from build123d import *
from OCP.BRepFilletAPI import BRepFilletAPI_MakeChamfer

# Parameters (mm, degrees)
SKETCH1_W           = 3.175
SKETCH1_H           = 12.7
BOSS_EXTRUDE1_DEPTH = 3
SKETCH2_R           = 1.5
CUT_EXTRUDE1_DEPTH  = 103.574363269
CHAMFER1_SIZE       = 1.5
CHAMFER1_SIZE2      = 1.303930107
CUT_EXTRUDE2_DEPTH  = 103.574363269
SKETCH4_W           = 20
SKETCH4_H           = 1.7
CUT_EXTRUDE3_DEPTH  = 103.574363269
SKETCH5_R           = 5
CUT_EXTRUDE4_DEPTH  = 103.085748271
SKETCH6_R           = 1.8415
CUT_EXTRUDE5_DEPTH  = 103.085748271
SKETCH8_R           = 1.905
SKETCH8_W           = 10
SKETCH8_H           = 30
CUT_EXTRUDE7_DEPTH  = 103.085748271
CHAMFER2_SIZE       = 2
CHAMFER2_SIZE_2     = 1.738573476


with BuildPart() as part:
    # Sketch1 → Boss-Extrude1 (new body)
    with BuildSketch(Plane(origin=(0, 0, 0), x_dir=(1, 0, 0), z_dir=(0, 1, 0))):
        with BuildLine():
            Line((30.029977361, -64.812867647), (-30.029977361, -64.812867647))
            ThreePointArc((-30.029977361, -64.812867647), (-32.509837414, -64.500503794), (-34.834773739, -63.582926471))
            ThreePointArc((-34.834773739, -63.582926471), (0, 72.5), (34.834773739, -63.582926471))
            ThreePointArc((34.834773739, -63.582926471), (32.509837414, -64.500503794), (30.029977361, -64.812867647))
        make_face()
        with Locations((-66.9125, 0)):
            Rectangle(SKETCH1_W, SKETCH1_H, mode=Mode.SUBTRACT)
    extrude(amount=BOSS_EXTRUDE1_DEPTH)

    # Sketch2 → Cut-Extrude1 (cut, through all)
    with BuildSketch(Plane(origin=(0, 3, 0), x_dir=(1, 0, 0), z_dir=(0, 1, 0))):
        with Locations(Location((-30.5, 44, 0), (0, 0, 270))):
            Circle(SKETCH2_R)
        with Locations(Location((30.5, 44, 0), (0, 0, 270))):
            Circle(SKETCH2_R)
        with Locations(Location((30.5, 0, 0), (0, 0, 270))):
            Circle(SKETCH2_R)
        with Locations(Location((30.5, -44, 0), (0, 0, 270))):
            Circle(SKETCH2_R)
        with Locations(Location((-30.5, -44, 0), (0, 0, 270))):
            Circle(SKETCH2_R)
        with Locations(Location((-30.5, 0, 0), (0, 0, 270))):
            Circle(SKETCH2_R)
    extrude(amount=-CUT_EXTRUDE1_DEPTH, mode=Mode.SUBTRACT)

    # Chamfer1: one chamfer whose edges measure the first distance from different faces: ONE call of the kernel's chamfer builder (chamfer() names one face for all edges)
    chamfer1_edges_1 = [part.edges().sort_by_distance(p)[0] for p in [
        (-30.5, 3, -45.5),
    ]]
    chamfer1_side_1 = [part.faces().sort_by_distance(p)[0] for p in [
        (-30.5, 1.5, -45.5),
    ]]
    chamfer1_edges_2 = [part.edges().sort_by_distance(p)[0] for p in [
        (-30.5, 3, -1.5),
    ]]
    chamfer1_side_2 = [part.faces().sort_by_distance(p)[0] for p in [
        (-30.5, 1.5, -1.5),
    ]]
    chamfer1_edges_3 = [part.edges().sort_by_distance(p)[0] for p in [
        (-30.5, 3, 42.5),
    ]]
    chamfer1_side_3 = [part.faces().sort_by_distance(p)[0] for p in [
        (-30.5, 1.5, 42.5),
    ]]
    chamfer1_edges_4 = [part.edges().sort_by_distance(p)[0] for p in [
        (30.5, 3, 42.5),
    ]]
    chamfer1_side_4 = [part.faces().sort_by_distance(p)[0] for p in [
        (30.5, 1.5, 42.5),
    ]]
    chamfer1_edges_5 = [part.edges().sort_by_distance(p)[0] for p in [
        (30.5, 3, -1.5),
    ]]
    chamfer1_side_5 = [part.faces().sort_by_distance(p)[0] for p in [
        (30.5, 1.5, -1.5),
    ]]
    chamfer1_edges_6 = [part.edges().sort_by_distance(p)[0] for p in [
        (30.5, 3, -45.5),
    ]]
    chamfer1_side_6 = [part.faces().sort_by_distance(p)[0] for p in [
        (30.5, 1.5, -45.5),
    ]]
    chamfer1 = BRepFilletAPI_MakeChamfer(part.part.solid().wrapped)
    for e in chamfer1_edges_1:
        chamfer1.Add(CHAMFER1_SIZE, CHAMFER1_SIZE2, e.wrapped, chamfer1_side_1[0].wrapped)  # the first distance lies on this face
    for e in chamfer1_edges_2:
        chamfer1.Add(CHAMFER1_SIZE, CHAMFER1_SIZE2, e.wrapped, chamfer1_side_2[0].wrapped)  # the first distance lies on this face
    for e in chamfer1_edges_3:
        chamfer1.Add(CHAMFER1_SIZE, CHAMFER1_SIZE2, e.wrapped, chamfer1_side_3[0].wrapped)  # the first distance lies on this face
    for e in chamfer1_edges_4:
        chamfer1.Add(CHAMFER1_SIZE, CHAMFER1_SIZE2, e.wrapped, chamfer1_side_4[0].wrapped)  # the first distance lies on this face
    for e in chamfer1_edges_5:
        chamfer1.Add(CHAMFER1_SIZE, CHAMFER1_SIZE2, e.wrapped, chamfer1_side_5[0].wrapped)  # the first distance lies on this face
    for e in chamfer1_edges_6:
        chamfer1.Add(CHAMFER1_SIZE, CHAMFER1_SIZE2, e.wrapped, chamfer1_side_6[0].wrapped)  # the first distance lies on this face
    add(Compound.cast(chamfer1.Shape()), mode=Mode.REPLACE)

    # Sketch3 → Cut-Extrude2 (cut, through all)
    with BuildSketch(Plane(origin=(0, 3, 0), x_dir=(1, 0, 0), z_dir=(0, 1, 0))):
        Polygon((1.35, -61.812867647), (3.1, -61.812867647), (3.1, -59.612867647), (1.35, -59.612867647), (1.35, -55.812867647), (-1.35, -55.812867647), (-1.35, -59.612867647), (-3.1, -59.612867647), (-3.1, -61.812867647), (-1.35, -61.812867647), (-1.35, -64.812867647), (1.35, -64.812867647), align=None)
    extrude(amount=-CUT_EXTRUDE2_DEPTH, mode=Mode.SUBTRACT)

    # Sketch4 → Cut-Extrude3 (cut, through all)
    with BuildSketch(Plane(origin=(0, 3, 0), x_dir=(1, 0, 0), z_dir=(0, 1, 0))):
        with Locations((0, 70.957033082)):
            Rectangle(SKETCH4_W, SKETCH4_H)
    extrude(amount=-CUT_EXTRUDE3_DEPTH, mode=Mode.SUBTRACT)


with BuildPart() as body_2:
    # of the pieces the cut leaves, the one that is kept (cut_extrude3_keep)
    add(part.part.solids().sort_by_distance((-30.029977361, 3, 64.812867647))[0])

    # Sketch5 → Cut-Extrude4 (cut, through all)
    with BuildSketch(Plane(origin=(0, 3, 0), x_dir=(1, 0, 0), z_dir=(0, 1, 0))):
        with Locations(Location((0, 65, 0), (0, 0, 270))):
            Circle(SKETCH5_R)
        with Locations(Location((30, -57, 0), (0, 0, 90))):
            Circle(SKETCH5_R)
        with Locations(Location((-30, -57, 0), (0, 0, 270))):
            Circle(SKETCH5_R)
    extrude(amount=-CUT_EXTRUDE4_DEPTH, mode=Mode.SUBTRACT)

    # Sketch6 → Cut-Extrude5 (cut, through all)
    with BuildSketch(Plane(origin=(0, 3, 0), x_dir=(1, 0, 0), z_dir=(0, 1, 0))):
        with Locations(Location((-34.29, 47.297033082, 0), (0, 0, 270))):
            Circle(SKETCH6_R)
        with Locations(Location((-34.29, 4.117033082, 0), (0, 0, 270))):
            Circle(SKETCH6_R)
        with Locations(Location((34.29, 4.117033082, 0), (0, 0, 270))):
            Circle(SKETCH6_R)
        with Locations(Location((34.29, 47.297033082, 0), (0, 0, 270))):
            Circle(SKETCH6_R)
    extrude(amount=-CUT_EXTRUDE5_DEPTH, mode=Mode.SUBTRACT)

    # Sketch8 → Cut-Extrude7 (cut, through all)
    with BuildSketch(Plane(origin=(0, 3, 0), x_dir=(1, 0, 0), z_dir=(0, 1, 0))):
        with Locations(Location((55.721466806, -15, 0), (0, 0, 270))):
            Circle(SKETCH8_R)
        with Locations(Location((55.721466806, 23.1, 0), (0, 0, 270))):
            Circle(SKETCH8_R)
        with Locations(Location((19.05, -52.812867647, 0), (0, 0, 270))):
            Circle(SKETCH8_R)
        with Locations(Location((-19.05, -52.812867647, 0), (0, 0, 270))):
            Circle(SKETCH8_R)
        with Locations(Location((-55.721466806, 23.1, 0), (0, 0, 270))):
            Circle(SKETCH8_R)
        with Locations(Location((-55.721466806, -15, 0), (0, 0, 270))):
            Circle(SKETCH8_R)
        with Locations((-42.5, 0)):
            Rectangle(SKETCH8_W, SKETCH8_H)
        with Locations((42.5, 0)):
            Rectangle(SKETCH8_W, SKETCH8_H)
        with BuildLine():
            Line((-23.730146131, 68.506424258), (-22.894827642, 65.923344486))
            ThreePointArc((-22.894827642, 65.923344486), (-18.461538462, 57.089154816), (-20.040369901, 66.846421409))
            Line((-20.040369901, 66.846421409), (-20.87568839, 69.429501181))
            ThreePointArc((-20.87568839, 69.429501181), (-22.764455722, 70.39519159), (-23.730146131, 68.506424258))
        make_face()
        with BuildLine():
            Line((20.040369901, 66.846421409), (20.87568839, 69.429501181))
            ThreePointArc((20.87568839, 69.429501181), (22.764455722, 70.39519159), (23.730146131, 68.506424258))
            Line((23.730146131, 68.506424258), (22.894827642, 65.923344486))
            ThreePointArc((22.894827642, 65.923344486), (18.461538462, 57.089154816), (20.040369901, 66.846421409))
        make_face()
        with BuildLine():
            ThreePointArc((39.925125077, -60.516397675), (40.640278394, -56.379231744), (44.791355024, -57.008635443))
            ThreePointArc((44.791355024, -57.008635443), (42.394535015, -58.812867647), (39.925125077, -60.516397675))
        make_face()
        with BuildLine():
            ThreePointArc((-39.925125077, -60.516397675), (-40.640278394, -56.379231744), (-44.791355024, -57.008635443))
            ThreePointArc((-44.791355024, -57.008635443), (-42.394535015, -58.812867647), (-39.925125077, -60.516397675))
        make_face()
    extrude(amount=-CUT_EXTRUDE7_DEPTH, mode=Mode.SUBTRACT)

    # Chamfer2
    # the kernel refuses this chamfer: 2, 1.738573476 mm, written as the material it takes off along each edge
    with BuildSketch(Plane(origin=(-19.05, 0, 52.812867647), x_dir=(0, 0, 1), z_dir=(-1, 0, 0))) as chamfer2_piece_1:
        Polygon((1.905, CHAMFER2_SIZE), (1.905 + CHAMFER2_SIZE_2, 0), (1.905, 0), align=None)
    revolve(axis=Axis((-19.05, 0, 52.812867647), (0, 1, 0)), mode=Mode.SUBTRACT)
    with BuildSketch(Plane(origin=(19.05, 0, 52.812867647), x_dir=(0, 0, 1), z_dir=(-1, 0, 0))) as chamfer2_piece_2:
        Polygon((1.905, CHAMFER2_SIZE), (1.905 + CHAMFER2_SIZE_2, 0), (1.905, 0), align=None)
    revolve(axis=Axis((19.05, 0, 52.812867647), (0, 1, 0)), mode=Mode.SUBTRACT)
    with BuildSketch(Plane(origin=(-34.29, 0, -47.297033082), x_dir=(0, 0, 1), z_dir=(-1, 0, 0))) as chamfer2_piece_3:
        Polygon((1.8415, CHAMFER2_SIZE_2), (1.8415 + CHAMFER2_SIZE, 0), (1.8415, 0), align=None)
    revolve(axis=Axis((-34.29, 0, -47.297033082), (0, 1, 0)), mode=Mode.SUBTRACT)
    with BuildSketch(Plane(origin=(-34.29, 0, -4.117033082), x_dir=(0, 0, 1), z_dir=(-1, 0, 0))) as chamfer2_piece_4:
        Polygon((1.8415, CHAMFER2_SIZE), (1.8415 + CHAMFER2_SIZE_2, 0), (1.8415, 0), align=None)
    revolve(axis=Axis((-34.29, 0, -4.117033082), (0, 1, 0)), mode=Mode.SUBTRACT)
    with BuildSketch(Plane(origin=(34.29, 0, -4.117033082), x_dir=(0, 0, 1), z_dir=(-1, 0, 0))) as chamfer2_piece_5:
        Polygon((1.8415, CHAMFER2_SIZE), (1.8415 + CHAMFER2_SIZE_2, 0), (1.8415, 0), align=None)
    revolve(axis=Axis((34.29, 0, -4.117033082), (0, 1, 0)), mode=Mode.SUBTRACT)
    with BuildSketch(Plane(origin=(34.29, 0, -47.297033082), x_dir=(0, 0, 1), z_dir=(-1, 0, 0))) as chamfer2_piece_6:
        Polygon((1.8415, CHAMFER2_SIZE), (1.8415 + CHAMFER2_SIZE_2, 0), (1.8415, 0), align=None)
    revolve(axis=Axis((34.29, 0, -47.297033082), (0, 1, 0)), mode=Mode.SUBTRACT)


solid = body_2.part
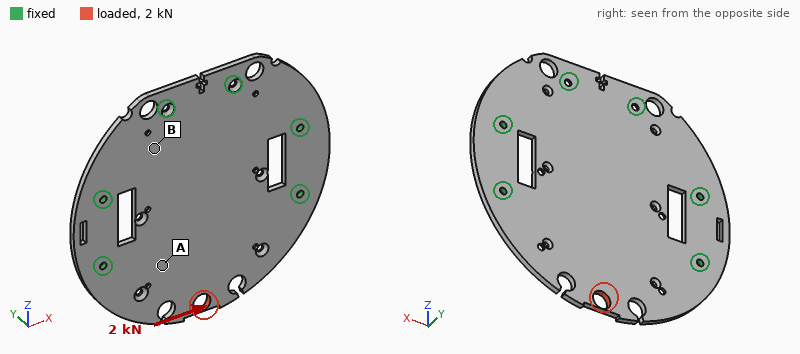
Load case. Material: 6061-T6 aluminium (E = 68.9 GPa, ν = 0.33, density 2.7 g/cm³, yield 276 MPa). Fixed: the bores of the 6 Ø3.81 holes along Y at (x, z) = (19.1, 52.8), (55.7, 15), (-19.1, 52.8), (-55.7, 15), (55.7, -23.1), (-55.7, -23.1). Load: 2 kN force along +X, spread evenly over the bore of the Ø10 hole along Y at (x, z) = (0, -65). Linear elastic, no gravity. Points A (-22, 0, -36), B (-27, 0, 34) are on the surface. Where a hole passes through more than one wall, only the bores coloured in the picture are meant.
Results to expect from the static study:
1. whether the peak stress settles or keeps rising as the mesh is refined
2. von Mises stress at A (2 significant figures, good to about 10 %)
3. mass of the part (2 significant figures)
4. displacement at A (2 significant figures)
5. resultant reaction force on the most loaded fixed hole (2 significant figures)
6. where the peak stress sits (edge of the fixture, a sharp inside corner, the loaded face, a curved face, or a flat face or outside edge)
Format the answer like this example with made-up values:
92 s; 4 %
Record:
keeps rising; 12 MPa; 120 g; 7.8 µm; 1.1 kN; a sharp inside corner
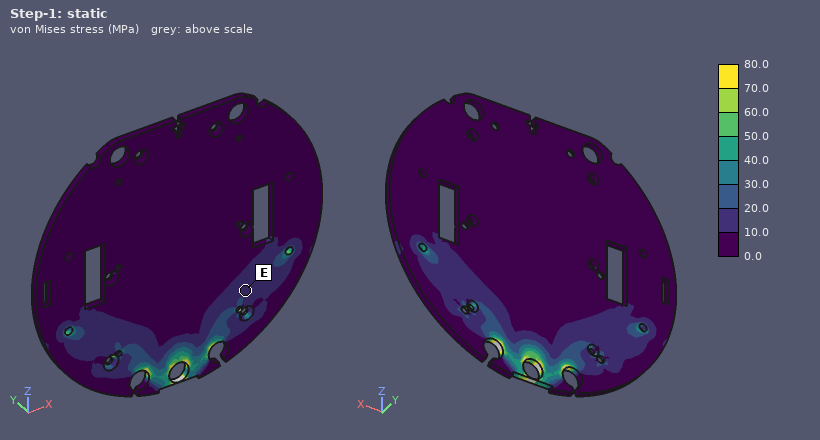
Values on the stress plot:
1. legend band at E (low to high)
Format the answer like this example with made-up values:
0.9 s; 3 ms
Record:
10.0 to 20.0 MPa
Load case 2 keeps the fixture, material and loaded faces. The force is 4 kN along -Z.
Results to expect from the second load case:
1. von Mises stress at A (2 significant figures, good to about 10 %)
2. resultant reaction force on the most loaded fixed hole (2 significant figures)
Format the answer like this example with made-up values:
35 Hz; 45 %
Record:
18 MPa; 890 N
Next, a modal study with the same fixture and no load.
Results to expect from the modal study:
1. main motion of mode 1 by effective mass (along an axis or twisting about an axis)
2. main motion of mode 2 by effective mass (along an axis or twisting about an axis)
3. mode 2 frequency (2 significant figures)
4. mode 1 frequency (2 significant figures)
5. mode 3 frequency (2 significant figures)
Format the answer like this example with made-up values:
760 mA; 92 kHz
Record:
along Y; along Y; 1600 Hz; 790 Hz; 2000 Hz
